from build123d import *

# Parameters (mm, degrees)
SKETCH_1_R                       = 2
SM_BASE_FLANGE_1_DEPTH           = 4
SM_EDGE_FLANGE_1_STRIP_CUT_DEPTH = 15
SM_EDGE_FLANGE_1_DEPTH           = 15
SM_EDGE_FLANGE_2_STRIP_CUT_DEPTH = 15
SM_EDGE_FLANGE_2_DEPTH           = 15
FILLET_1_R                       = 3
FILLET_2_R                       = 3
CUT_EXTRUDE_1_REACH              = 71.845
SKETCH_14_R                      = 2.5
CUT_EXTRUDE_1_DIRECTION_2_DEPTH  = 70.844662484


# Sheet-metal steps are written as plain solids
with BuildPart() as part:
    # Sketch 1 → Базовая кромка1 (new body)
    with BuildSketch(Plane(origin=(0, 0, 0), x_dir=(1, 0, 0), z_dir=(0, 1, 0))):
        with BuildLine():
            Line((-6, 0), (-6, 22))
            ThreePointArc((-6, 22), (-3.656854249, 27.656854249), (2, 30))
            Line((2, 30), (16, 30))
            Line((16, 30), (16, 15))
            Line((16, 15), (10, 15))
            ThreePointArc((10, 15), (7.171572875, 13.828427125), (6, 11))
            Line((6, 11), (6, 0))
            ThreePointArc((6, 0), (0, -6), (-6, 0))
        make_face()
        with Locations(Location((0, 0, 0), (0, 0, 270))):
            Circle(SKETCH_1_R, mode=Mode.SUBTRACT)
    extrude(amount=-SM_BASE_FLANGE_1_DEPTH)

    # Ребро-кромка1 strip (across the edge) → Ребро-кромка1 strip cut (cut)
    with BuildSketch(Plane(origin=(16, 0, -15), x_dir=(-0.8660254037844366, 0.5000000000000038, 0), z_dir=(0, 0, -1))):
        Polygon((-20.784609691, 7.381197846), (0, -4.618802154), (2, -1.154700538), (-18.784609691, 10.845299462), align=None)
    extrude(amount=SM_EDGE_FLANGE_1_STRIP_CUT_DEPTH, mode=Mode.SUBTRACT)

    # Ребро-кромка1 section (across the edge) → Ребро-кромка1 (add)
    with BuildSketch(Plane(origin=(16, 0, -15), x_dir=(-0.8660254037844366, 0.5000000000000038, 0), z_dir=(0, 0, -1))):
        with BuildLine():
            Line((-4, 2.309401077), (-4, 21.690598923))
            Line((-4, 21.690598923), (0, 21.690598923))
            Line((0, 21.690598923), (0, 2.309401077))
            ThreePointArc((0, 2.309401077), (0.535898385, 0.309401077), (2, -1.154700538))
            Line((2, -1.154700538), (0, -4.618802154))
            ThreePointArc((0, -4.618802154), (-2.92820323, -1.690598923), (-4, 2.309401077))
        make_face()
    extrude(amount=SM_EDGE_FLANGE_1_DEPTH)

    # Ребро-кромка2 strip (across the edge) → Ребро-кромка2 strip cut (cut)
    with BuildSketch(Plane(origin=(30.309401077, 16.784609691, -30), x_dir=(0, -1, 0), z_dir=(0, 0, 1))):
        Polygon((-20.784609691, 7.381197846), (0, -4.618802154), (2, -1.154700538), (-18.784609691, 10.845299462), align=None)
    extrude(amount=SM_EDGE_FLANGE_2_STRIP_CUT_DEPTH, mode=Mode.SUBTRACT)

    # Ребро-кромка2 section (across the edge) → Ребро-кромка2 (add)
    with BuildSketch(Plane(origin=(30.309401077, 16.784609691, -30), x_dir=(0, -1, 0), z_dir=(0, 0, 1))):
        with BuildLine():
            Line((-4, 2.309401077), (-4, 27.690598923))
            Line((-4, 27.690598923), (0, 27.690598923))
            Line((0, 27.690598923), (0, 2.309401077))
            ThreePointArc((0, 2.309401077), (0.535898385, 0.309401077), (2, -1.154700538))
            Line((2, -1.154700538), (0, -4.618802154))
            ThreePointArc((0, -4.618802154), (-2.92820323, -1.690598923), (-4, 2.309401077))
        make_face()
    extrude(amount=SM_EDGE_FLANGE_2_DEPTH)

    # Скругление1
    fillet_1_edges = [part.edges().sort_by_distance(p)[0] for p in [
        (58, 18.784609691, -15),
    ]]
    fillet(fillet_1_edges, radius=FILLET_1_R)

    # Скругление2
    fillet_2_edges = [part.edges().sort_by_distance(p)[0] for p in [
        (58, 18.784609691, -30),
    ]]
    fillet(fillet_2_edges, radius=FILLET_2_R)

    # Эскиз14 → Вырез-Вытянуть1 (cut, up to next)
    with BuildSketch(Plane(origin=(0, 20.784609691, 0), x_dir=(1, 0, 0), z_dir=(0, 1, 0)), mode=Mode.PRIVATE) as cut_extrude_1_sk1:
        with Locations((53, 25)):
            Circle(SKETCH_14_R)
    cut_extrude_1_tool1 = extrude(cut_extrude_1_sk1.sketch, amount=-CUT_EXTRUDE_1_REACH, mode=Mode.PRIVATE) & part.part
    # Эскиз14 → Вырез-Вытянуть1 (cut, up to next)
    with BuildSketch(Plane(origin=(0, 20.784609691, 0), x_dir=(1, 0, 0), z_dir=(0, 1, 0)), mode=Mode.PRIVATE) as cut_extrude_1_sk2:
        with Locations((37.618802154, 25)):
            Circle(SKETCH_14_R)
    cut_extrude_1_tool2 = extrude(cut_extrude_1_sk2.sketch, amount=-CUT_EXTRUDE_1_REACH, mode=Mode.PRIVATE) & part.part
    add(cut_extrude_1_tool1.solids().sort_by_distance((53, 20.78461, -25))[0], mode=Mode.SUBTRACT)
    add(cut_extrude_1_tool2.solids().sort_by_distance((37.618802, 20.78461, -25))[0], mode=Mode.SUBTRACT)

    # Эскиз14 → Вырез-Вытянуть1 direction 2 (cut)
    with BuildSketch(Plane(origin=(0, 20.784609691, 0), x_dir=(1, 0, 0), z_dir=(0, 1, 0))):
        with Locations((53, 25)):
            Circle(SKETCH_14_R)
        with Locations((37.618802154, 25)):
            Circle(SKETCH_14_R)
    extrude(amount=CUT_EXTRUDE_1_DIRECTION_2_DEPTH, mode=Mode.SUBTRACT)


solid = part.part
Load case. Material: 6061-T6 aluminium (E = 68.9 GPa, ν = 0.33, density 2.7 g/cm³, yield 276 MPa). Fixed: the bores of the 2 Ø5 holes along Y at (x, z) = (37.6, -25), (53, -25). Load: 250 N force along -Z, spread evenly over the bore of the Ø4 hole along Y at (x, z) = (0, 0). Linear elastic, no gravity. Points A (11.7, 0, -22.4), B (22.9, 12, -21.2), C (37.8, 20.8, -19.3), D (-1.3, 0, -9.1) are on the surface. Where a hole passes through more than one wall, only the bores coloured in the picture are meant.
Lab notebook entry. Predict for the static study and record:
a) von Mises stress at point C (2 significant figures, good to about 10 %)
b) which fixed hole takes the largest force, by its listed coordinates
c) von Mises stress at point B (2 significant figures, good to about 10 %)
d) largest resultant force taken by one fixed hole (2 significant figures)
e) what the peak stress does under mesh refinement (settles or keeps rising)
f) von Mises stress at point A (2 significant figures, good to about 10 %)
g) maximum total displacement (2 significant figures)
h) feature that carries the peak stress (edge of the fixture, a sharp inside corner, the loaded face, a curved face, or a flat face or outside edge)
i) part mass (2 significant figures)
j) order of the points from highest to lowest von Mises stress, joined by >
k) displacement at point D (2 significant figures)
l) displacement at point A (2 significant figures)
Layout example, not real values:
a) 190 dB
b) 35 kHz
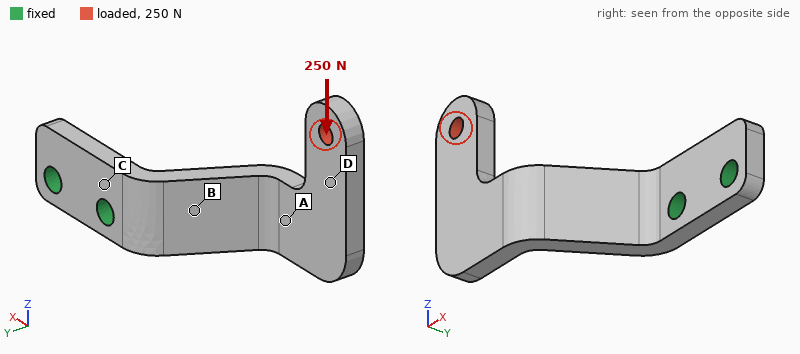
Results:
a) 68 MPa
b) (37.6, -25)
c) 92 MPa
d) 600 N
e) keeps rising
f) 25 MPa
g) 0.44 mm
h) edge of the fixture
i) 14 g
j) B > C > A > D
k) 0.34 mm
l) 0.17 mm
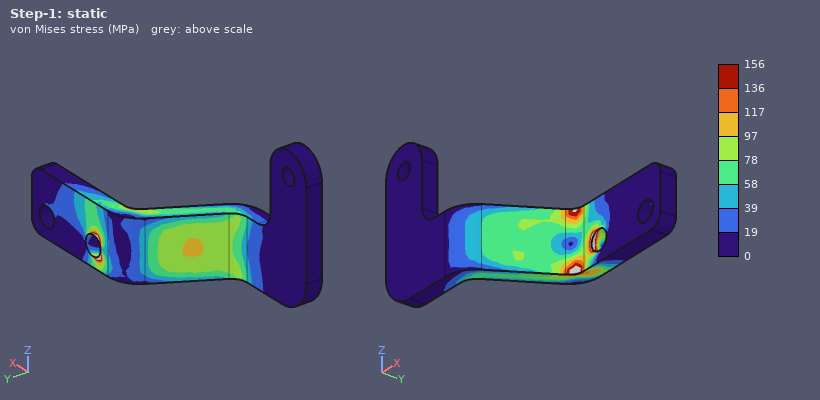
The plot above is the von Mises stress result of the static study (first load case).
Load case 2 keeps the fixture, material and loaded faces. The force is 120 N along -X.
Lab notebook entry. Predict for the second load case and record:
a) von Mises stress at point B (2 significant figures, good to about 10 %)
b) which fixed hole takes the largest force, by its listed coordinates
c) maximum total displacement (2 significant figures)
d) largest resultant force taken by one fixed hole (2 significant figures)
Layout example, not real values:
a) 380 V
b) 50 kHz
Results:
a) 66 MPa
b) (53, -25)
c) 0.55 mm
d) 140 N
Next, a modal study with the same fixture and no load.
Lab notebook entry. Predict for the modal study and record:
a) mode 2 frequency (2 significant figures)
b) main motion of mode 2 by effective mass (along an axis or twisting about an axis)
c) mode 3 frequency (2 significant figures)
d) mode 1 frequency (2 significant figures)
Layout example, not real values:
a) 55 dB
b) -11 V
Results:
a) 1900 Hz
b) along Z
c) 2900 Hz
d) 930 Hz
